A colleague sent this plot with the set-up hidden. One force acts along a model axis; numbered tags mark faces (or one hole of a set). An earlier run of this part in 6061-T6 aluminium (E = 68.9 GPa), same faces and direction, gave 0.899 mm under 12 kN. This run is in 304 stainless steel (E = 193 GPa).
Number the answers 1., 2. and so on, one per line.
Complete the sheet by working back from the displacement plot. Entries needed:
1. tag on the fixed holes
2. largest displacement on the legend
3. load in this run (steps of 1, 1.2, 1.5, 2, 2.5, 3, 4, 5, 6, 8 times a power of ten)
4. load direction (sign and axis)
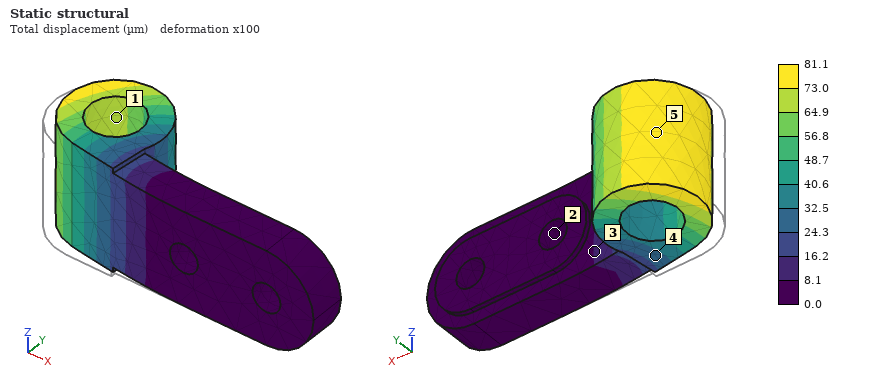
1. 2
2. 81.1 µm
3. 3 kN
4. +Y
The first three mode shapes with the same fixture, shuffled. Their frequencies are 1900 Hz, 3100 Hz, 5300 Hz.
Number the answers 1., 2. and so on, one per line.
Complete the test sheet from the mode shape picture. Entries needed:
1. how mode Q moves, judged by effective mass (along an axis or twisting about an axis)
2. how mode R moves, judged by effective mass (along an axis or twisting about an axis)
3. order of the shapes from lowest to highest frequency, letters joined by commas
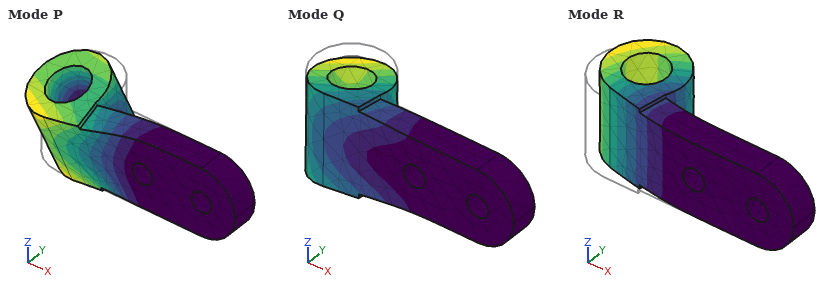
1. along Z
2. along Y
3. R, Q, P
